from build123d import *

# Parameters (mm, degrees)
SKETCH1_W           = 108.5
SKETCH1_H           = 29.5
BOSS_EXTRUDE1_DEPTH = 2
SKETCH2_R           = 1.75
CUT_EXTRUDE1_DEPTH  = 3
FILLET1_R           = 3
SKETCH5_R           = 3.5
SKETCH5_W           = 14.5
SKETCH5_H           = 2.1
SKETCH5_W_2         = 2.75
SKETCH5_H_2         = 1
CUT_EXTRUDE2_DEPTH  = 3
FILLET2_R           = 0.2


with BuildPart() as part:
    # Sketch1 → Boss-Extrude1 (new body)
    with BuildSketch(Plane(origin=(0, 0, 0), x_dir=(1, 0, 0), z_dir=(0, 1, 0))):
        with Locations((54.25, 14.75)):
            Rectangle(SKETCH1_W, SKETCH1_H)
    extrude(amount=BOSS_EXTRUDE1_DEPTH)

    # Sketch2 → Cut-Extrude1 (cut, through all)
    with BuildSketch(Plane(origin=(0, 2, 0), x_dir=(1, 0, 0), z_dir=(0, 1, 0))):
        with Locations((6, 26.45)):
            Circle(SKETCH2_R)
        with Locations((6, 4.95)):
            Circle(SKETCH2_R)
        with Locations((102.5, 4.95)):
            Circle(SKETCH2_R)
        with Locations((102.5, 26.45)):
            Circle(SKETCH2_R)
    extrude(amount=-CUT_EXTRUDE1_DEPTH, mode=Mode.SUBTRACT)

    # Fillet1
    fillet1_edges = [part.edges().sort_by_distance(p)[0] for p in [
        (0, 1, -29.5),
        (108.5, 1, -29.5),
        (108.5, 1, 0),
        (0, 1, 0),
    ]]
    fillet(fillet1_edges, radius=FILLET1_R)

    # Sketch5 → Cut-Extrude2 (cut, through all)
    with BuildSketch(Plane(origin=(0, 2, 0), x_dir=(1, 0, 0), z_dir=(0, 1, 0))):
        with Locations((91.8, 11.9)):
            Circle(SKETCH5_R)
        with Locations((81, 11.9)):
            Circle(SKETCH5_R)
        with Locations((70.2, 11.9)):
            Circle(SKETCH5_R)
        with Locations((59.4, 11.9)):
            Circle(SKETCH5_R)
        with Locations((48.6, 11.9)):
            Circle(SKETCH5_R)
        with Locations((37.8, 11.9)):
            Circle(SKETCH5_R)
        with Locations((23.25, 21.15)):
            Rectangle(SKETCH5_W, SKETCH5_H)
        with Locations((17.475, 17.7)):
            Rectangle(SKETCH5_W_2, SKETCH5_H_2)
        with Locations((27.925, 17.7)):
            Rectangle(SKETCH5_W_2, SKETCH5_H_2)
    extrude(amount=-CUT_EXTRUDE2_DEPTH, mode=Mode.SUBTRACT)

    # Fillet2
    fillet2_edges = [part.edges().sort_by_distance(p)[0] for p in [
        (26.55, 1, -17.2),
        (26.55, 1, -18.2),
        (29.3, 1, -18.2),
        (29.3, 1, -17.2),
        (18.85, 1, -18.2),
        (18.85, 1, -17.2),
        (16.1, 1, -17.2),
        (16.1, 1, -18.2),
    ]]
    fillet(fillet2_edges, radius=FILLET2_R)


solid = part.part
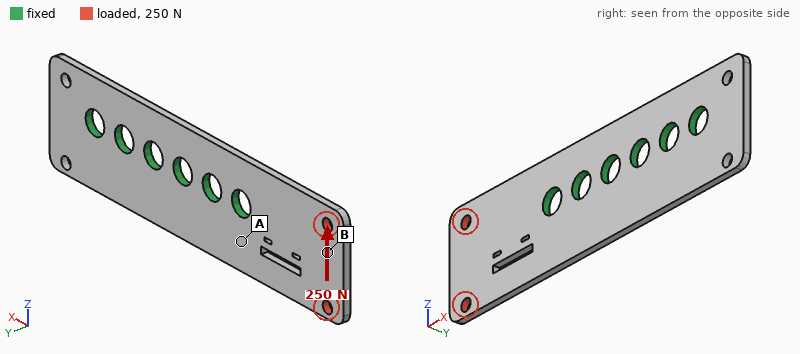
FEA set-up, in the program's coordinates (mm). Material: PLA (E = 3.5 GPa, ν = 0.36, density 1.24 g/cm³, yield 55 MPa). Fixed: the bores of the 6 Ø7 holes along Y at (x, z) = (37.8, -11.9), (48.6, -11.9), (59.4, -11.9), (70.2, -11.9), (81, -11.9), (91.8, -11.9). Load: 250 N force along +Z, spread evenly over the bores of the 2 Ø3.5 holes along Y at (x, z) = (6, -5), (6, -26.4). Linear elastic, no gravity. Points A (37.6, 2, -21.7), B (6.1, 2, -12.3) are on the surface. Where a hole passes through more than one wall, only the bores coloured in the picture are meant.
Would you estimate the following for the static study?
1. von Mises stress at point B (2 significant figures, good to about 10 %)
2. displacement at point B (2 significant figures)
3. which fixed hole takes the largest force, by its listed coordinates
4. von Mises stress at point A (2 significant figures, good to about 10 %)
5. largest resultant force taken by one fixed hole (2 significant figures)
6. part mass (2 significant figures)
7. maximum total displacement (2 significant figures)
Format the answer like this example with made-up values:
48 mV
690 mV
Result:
5.3 MPa
0.51 mm
(37.8, -11.9)
11 MPa
470 N
7.2 g
0.64 mm
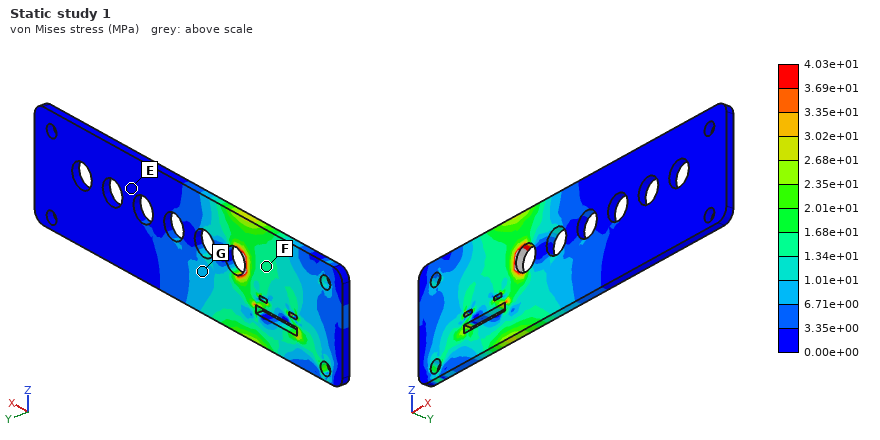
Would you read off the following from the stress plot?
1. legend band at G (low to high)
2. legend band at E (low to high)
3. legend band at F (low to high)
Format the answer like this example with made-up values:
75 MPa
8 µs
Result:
6.71e+00 to 1.01e+01 MPa
0.00e+00 to 3.35e+00 MPa
1.34e+01 to 1.68e+01 MPa
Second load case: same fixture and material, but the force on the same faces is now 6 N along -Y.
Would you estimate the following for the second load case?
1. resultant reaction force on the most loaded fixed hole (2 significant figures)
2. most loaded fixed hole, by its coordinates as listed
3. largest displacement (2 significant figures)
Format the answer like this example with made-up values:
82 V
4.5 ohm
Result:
9.1 N
(37.8, -11.9)
1.1 mm
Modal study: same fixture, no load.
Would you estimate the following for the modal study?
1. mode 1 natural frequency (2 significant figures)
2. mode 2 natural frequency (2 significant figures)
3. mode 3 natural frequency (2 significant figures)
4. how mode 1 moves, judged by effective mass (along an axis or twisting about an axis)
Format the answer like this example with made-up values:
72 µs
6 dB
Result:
420 Hz
1000 Hz
2000 Hz
along Y
